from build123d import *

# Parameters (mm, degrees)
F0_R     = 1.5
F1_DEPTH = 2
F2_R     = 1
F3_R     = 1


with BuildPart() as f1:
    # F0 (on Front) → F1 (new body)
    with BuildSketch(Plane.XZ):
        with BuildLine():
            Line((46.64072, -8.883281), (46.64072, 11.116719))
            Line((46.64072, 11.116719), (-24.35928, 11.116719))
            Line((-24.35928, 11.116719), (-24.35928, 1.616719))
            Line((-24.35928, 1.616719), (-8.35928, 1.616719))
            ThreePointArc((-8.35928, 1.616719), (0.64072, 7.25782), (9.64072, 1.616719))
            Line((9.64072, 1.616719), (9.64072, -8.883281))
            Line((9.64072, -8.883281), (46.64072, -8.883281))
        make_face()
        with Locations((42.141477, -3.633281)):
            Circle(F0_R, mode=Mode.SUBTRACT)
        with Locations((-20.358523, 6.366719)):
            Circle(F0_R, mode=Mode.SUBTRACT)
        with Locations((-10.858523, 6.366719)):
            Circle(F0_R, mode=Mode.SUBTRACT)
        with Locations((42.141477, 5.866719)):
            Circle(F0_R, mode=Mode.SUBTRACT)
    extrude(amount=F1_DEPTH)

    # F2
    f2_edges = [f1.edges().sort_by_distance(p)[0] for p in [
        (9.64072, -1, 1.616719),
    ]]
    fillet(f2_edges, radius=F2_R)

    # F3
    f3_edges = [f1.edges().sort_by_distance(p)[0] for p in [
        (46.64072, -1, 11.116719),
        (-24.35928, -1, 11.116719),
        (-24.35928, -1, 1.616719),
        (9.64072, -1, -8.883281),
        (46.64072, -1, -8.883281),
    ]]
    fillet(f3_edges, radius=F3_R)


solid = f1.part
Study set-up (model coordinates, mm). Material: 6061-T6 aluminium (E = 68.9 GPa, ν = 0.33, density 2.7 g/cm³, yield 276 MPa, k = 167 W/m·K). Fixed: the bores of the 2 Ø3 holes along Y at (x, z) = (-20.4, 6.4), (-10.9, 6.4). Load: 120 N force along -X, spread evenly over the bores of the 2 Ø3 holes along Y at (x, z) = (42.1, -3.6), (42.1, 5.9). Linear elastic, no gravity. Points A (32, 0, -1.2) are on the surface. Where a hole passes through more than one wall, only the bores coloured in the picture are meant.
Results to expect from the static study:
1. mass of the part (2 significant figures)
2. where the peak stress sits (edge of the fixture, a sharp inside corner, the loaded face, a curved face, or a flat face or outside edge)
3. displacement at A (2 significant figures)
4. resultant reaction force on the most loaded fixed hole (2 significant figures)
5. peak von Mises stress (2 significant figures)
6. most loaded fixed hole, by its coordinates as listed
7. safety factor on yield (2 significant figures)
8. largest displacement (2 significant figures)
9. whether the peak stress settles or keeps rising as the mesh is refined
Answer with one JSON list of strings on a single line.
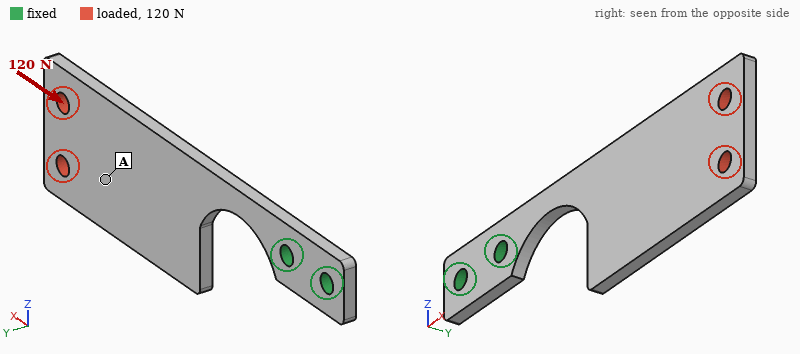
["5.2 g", "a curved face", "0.51 mm", "130 N", "230 MPa", "(-10.9, 6.4)", "1.2", "0.76 mm", "settles"]
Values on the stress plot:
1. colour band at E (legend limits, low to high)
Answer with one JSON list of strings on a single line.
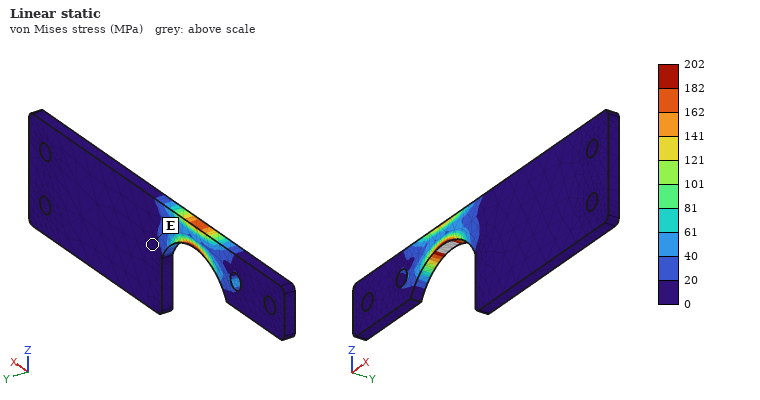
["0 to 20 MPa"]
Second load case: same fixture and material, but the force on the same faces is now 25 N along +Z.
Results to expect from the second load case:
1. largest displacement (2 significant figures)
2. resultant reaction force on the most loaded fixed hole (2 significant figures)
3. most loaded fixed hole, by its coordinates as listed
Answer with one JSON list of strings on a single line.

["0.88 mm", "94 N", "(-10.9, 6.4)"]
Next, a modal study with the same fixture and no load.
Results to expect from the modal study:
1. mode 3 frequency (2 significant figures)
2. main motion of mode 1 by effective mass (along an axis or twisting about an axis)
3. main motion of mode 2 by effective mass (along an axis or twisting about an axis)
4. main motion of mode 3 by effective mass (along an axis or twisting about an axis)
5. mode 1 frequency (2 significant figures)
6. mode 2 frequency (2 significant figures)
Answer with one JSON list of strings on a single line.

["1300 Hz", "along Y", "along Z", "twisting about X", "270 Hz", "630 Hz"]
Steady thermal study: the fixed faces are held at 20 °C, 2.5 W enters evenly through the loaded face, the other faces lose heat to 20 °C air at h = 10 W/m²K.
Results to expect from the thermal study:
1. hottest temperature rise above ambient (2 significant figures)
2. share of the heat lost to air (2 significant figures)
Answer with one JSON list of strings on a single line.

["37 K", "22 %"]
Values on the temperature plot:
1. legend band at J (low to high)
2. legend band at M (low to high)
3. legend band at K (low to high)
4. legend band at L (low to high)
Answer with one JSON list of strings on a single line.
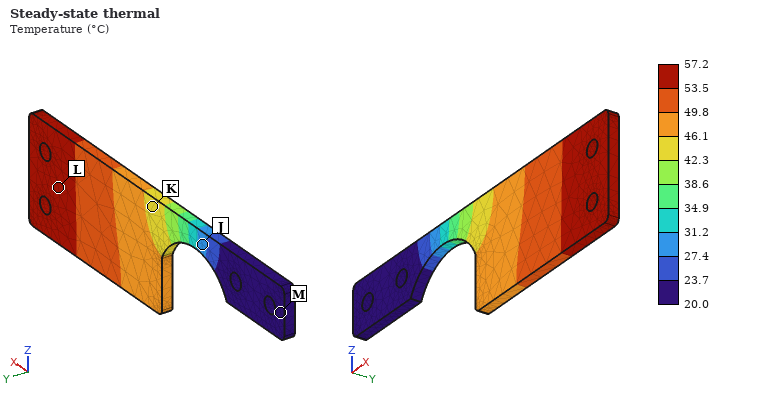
["27.4 to 31.2 °C", "20.0 to 23.7 °C", "42.3 to 46.1 °C", "53.5 to 57.2 °C"]
